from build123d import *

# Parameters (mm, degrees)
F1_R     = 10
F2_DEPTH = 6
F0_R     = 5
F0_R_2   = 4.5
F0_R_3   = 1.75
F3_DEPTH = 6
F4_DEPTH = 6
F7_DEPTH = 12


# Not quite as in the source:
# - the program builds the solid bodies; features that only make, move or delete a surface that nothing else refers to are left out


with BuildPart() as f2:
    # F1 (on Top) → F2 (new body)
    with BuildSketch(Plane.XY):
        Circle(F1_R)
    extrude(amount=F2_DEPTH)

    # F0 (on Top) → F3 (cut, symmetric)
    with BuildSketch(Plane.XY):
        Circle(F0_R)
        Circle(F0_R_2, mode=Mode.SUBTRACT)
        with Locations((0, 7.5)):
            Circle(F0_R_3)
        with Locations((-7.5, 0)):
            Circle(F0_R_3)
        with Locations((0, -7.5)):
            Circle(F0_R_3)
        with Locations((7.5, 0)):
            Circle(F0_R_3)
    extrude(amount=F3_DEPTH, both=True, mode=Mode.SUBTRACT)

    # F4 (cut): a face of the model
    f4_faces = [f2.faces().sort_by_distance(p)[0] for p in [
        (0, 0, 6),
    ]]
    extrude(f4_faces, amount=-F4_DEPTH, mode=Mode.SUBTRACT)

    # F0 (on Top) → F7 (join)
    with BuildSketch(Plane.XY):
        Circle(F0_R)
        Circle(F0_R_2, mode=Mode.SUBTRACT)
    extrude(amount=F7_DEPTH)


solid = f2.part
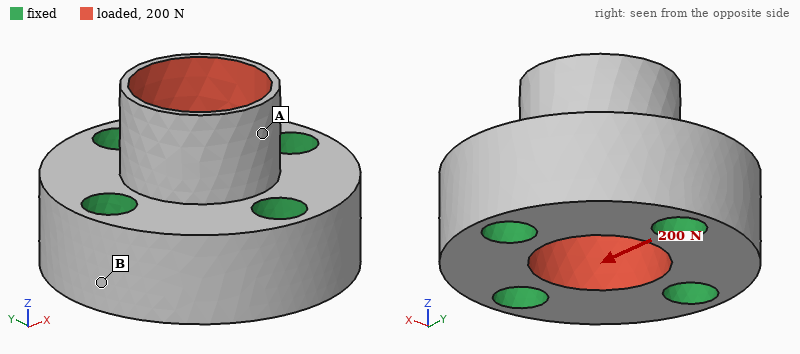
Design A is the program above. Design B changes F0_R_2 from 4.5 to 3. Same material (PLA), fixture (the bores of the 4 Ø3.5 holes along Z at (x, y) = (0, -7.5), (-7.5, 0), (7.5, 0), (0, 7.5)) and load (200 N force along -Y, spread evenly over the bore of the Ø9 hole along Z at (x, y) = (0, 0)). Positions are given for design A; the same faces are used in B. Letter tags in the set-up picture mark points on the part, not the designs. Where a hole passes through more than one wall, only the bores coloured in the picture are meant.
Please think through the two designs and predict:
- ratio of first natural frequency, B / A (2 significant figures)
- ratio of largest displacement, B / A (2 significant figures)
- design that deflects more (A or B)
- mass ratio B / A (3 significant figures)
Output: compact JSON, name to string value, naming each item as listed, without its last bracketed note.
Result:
{"ratio of first natural frequency, B / A": "1.5", "ratio of largest displacement, B / A": "0.34", "design that deflects more": "A", "mass ratio B / A": "1.31"}
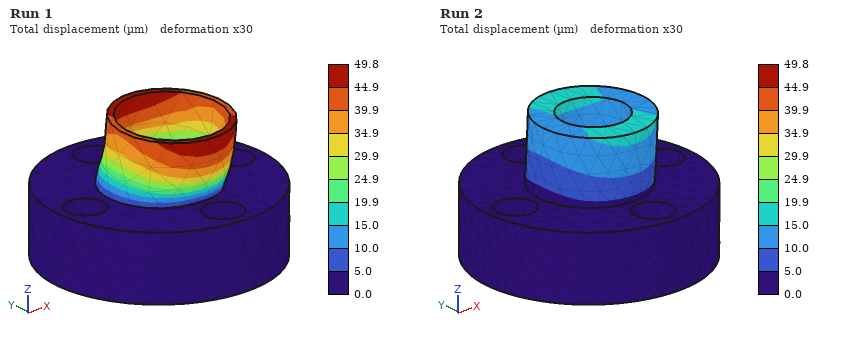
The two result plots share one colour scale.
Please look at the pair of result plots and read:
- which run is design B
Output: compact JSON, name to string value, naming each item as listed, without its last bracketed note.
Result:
{"which run is design B": "Run 2"}
